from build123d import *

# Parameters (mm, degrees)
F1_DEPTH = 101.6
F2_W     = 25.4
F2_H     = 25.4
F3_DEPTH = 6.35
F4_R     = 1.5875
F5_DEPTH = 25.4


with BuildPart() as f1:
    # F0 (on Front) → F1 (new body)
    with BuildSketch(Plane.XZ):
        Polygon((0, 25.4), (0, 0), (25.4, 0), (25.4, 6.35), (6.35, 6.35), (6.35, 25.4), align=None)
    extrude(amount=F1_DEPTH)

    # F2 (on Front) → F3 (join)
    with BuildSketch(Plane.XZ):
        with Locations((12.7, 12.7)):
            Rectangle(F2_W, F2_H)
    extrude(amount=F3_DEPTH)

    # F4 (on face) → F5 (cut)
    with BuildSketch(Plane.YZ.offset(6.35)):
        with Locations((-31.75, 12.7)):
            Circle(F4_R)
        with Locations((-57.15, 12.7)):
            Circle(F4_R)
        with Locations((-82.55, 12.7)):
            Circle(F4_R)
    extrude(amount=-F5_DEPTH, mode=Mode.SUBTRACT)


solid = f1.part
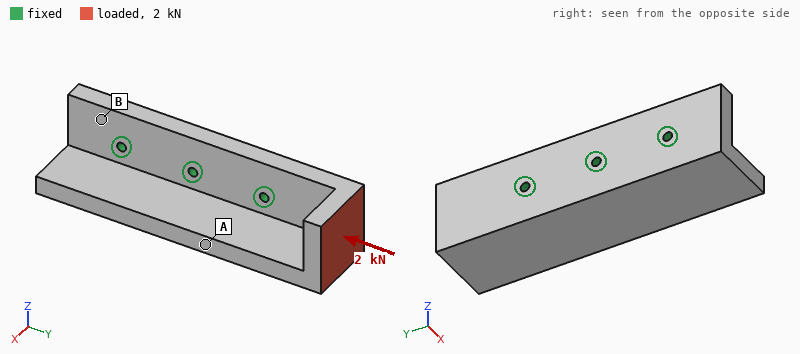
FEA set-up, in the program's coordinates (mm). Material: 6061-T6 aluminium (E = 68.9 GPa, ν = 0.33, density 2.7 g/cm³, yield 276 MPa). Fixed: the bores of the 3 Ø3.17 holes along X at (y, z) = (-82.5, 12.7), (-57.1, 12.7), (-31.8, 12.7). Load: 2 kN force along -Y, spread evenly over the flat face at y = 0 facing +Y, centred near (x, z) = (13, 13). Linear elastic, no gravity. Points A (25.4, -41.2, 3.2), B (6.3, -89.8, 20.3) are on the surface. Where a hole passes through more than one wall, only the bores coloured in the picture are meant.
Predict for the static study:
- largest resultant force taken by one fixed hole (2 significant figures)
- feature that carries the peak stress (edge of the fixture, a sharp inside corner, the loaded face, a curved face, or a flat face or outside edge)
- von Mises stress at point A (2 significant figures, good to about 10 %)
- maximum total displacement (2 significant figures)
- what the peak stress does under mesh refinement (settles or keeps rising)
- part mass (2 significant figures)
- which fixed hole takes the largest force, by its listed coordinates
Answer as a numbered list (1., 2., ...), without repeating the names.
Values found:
1. 1.2 kN
2. edge of the fixture
3. 15 MPa
4. 76 µm
5. keeps rising
6. 83 g
7. (-31.8, 12.7)
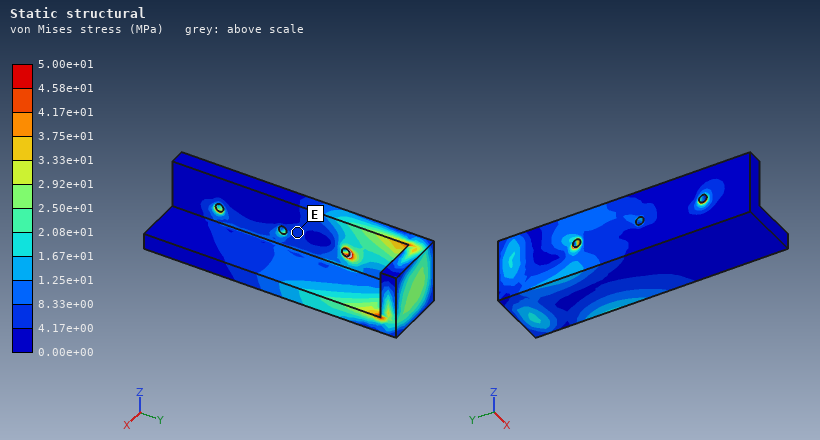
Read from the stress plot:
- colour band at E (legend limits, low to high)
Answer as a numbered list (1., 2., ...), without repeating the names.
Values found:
1. 4.17e+00 to 8.33e+00 MPa
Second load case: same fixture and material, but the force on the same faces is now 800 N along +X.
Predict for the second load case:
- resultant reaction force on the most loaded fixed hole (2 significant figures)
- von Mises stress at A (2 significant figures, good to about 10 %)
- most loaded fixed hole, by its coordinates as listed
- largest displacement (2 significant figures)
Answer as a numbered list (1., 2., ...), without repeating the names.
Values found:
1. 1.4 kN
2. 20 MPa
3. (-31.8, 12.7)
4. 70 µm
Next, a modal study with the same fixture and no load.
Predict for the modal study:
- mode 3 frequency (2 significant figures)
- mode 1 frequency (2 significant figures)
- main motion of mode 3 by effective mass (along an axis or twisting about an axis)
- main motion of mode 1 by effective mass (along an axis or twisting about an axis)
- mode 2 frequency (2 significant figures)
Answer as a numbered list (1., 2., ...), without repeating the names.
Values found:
1. 6100 Hz
2. 4000 Hz
3. along X
4. along Z
5. 5100 Hz
